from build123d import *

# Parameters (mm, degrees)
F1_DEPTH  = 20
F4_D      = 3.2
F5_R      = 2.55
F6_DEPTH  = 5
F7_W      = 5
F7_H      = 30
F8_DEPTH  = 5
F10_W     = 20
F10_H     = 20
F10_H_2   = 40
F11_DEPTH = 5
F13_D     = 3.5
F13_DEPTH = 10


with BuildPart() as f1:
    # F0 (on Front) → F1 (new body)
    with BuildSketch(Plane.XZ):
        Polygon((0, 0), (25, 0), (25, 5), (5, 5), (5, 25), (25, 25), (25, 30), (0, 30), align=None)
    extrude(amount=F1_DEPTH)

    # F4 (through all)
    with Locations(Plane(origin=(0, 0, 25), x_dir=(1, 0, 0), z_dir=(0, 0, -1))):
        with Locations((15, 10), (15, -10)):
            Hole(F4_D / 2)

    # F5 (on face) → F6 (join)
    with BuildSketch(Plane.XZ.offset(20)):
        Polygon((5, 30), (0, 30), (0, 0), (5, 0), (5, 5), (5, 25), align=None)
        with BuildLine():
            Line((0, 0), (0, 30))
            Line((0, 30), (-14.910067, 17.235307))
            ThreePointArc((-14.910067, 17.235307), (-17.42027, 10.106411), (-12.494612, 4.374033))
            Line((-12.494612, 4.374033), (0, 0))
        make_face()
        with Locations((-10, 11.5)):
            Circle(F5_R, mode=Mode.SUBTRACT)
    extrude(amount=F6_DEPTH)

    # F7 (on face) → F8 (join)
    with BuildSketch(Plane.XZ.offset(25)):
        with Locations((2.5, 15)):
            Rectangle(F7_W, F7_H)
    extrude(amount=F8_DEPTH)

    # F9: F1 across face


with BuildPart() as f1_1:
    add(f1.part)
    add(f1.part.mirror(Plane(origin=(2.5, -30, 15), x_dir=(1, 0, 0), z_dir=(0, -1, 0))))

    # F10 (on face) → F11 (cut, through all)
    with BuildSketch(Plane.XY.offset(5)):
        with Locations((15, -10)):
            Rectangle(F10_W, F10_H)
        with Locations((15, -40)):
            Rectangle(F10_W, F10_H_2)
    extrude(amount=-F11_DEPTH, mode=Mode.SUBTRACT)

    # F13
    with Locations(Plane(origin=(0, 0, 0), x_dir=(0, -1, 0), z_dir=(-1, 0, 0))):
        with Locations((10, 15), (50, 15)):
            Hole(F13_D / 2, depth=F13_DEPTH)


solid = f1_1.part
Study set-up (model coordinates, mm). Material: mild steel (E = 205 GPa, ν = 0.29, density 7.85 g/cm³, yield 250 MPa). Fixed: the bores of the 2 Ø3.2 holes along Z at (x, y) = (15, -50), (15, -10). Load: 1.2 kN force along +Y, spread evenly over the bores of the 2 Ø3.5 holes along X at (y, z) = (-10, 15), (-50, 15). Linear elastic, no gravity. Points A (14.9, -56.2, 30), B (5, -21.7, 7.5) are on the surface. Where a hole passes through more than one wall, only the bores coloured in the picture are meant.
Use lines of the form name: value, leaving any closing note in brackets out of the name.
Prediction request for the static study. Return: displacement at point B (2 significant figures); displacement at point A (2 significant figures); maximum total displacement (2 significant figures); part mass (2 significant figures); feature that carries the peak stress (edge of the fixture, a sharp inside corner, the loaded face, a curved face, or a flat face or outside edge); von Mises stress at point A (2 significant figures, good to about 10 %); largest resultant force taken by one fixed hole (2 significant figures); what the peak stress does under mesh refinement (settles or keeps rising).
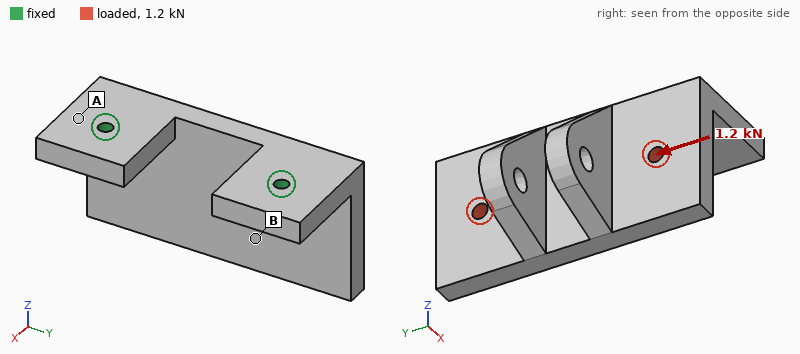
displacement at point B: 9.3 µm
displacement at point A: 2.2 µm
maximum total displacement: 13 µm
part mass: 130 g
feature that carries the peak stress: edge of the fixture
von Mises stress at point A: 21 MPa
largest resultant force taken by one fixed hole: 720 N
what the peak stress does under mesh refinement: keeps rising
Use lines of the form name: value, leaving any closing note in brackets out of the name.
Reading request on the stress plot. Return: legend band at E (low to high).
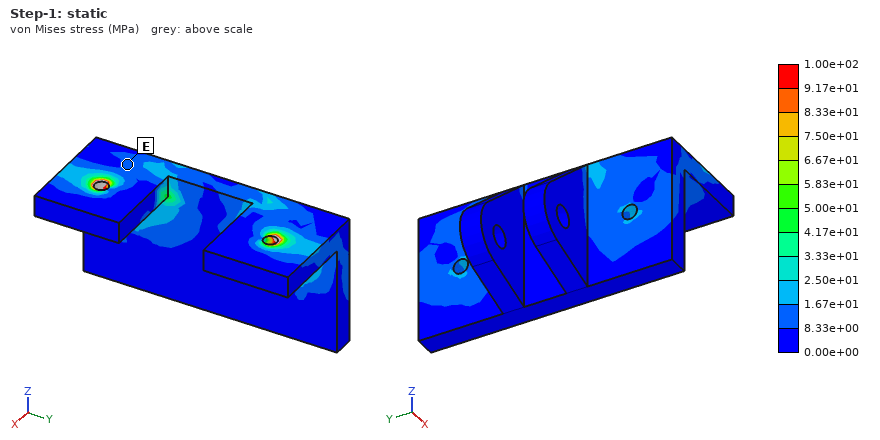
legend band at E: 8.33e+00 to 1.67e+01 MPa
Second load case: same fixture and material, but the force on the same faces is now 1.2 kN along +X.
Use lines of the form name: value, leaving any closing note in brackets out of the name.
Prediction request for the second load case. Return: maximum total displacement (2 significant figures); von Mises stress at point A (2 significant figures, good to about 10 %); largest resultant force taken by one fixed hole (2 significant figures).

maximum total displacement: 85 µm
von Mises stress at point A: 40 MPa
largest resultant force taken by one fixed hole: 600 N
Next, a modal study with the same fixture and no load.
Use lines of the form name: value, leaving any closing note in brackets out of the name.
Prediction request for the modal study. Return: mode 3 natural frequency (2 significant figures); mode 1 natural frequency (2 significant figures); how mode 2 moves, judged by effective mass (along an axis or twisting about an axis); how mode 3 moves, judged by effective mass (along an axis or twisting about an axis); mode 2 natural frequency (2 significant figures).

mode 3 natural frequency: 6800 Hz
mode 1 natural frequency: 2000 Hz
how mode 2 moves, judged by effective mass: along Y
how mode 3 moves, judged by effective mass: along Y
mode 2 natural frequency: 5100 Hz
